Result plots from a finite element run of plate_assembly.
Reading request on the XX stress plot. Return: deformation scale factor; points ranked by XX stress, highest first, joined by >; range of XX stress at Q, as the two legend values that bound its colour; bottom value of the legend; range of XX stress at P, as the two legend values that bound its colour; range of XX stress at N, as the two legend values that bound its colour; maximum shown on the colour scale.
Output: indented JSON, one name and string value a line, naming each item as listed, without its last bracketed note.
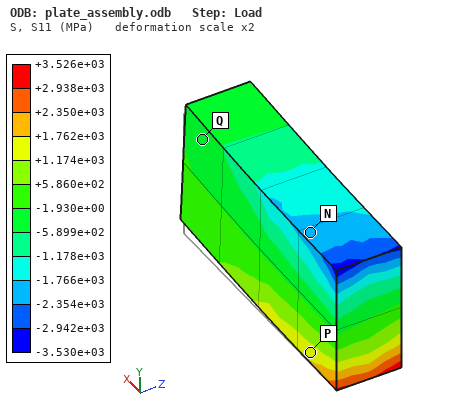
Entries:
{
  "deformation scale factor": "2",
  "points ranked by XX stress, highest first, joined by >": "P > Q > N",
  "range of XX stress at Q, as the two legend values that bound its colour": "-5.899e+02 to -1.930e+00 MPa",
  "bottom value of the legend": "-3.530e+03 MPa",
  "range of XX stress at P, as the two legend values that bound its colour": "+1.174e+03 to +1.762e+03 MPa",
  "range of XX stress at N, as the two legend values that bound its colour": "-2.354e+03 to -1.766e+03 MPa",
  "maximum shown on the colour scale": "+3.526e+03 MPa"
}
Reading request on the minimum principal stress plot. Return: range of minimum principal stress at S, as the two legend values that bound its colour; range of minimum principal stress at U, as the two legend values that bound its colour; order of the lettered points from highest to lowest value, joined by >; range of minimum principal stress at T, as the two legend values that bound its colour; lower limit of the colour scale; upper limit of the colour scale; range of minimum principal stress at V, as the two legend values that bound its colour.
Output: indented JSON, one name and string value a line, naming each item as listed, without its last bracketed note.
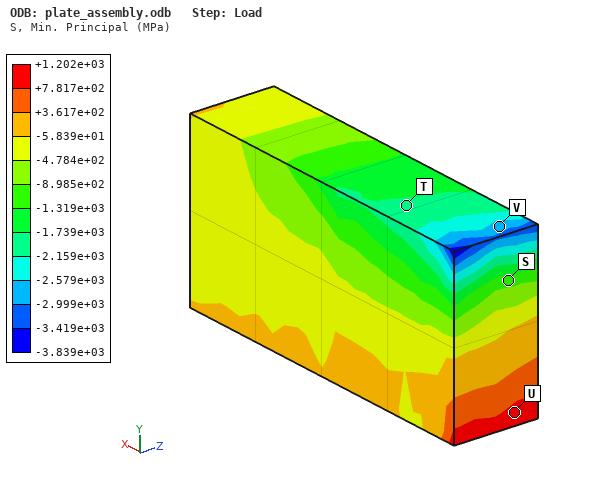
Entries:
{
  "range of minimum principal stress at S, as the two legend values that bound its colour": "-1.319e+03 to -8.985e+02 MPa",
  "range of minimum principal stress at U, as the two legend values that bound its colour": "+7.817e+02 to +1.202e+03 MPa",
  "order of the lettered points from highest to lowest value, joined by >": "U > S > T > V",
  "range of minimum principal stress at T, as the two legend values that bound its colour": "-2.159e+03 to -1.739e+03 MPa",
  "lower limit of the colour scale": "-3.839e+03 MPa",
  "upper limit of the colour scale": "+1.202e+03 MPa",
  "range of minimum principal stress at V, as the two legend values that bound its colour": "-2.999e+03 to -2.579e+03 MPa"
}
